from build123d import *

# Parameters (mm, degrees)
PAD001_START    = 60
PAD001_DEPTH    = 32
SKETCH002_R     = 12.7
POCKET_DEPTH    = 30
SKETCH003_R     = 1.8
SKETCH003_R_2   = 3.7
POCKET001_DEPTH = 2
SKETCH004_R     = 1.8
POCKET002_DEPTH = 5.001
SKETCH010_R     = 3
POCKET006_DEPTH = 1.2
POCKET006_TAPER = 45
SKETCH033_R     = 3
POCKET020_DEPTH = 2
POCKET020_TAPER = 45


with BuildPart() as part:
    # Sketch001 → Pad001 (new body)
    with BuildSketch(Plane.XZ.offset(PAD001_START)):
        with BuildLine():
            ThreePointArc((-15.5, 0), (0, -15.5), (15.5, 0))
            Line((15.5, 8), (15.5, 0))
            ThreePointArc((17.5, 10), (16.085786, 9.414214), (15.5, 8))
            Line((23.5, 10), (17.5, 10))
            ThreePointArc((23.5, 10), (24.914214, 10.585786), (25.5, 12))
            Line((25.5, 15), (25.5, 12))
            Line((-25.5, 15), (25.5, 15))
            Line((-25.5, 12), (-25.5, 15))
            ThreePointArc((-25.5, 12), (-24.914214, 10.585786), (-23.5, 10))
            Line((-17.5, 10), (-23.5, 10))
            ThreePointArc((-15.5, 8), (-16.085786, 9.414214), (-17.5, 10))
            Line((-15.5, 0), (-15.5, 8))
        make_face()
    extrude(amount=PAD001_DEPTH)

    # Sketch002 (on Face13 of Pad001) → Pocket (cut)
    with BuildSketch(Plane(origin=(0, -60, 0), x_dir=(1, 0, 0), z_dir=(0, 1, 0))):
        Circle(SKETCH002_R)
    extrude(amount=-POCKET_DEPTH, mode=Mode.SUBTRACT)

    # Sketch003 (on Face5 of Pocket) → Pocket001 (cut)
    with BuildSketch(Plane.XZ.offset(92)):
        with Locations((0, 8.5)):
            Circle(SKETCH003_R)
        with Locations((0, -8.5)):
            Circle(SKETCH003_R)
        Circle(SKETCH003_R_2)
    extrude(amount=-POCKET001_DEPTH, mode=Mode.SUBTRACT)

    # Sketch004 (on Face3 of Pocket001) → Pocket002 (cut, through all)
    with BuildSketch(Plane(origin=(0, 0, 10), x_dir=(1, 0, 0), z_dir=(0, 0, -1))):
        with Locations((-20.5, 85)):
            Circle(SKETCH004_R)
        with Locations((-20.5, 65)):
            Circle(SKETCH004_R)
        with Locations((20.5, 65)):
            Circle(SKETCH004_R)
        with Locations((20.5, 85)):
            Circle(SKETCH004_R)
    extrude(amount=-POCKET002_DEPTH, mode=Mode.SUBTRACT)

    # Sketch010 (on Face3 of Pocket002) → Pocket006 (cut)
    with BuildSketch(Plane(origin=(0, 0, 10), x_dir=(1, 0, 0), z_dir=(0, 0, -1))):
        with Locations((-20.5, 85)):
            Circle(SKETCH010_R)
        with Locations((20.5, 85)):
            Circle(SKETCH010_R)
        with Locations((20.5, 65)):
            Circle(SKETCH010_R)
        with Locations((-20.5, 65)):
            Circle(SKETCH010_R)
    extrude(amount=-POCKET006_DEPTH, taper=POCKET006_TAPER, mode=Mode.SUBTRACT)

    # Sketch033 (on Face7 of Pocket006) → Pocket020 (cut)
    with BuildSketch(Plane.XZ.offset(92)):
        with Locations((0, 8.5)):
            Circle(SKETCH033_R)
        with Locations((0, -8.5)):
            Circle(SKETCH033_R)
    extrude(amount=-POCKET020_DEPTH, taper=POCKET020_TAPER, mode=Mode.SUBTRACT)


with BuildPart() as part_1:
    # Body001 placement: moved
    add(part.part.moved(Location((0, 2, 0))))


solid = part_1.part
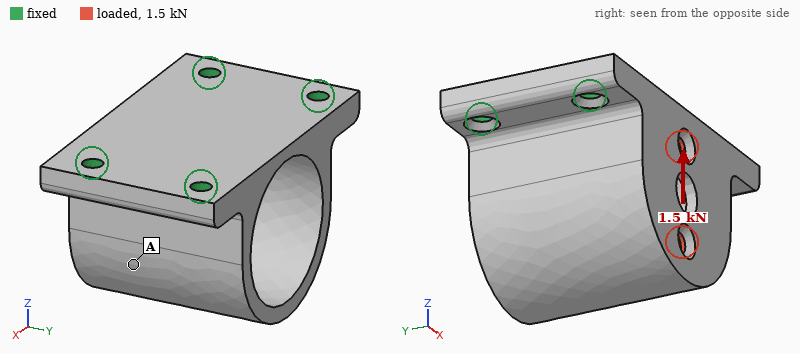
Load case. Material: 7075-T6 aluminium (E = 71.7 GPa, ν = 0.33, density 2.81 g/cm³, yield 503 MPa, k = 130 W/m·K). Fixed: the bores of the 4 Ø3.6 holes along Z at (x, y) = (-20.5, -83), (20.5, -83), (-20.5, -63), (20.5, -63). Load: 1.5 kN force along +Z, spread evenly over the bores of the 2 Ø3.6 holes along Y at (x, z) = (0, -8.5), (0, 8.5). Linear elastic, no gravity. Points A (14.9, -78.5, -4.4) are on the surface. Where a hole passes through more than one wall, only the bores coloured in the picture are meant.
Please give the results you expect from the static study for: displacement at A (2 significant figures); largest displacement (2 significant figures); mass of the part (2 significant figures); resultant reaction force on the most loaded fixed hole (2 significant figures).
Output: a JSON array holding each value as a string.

["11 µm", "25 µm", "41 g", "960 N"]
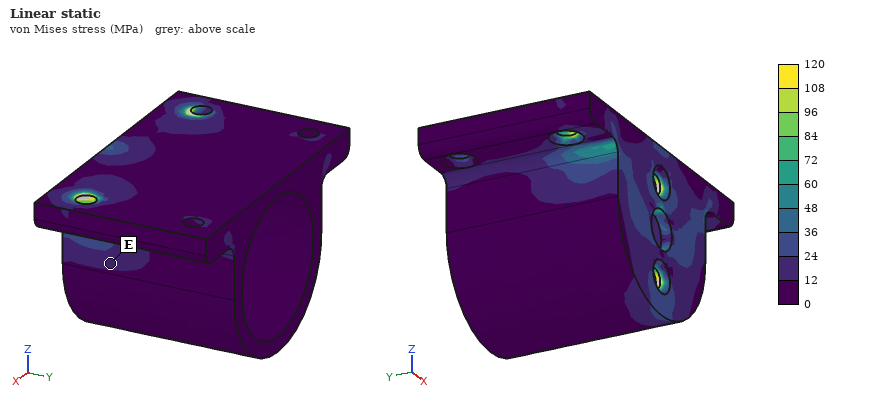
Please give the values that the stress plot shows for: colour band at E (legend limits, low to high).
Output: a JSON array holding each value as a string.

["12 to 24 MPa"]
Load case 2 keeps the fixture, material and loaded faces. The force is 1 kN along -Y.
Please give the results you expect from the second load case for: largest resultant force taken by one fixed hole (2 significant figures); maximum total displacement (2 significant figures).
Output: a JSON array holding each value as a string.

["450 N", "47 µm"]
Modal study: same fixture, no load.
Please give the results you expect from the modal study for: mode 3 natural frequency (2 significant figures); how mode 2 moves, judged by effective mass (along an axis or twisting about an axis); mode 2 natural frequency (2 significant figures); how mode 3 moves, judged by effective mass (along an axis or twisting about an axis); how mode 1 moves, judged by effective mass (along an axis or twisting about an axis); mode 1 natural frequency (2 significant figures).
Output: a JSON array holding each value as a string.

["13 kHz", "along Y", "9700 Hz", "along Z", "along X", "8400 Hz"]
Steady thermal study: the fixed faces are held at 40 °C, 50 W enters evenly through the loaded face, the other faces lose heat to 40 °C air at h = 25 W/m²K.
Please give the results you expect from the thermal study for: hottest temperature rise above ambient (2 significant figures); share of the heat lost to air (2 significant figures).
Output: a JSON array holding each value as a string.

["73 K", "7.4 %"]
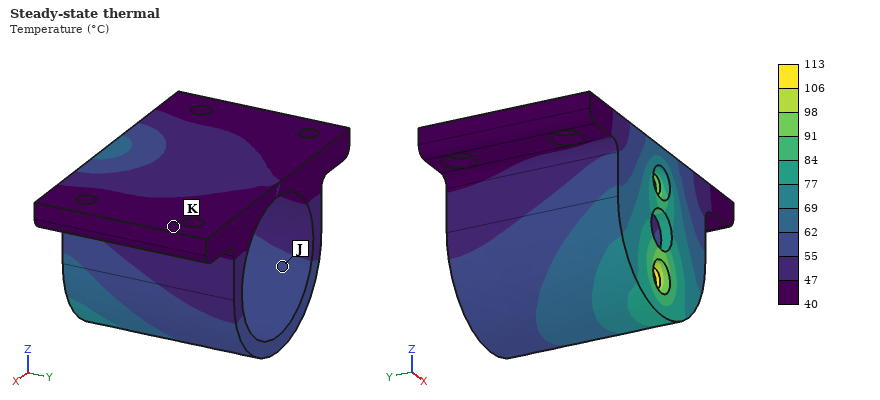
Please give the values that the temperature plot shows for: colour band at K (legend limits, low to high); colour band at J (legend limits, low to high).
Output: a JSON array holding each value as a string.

["40 to 47 °C", "55 to 62 °C"]
